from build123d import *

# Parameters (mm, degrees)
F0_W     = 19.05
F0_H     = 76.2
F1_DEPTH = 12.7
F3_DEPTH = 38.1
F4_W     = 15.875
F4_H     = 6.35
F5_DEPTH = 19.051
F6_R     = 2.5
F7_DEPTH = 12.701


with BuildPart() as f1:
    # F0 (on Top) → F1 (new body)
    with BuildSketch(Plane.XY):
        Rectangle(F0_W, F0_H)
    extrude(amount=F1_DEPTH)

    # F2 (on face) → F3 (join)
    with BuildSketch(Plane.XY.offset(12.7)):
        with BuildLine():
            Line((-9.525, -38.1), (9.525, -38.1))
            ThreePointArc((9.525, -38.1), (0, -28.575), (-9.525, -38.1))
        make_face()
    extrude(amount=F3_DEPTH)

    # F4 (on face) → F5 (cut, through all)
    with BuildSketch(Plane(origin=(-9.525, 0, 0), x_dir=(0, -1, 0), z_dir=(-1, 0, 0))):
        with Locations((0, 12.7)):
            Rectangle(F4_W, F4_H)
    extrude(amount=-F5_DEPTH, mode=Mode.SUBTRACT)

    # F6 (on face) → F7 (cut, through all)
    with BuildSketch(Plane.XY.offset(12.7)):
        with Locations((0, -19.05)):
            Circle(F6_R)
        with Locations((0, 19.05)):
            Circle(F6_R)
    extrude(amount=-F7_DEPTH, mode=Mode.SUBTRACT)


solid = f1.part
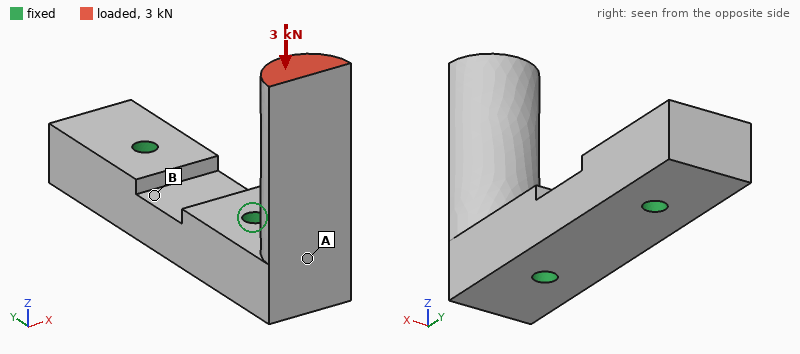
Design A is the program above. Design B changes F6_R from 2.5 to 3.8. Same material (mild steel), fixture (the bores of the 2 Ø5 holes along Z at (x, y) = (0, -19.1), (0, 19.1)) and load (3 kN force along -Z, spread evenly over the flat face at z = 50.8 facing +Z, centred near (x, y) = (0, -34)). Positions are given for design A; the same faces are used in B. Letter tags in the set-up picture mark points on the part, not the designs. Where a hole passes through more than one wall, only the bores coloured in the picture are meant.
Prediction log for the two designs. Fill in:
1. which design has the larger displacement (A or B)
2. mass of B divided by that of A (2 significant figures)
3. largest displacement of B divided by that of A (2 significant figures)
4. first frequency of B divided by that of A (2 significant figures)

A
0.97
0.81
1.0
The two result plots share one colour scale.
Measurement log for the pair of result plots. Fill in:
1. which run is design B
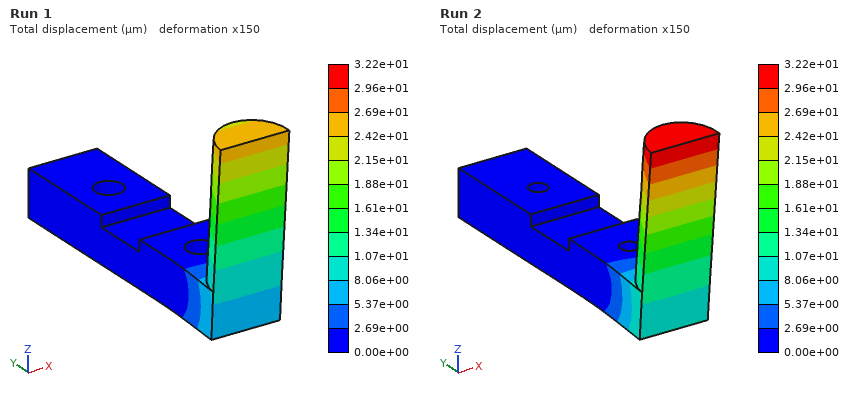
Run 1
